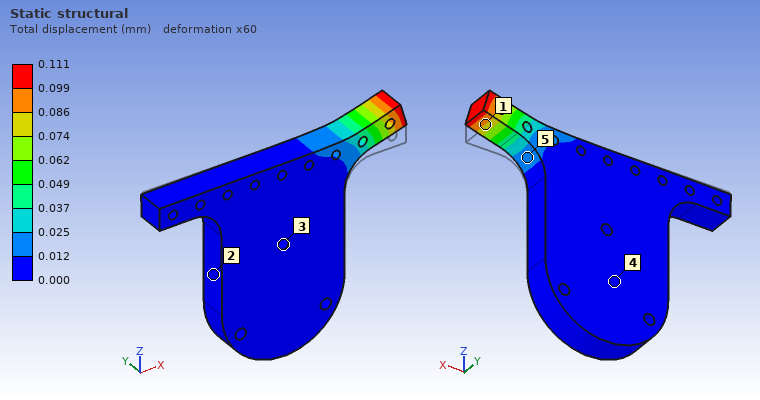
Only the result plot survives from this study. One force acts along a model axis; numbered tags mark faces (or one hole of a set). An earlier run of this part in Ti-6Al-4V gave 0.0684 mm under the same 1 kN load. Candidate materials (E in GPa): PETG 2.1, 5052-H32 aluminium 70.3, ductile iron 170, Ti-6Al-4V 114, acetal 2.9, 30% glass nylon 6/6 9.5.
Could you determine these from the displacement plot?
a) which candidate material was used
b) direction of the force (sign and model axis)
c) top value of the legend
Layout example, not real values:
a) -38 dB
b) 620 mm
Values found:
a) 5052-H32 aluminium
b) +Z
c) 0.111 mm
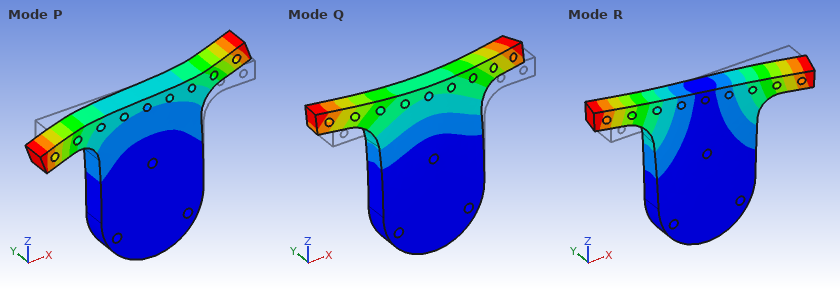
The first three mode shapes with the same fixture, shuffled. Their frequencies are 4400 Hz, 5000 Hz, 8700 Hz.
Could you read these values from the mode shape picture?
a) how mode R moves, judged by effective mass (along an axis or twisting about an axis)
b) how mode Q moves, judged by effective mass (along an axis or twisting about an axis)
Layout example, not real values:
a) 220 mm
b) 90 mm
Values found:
a) twisting about Z
b) along Y
